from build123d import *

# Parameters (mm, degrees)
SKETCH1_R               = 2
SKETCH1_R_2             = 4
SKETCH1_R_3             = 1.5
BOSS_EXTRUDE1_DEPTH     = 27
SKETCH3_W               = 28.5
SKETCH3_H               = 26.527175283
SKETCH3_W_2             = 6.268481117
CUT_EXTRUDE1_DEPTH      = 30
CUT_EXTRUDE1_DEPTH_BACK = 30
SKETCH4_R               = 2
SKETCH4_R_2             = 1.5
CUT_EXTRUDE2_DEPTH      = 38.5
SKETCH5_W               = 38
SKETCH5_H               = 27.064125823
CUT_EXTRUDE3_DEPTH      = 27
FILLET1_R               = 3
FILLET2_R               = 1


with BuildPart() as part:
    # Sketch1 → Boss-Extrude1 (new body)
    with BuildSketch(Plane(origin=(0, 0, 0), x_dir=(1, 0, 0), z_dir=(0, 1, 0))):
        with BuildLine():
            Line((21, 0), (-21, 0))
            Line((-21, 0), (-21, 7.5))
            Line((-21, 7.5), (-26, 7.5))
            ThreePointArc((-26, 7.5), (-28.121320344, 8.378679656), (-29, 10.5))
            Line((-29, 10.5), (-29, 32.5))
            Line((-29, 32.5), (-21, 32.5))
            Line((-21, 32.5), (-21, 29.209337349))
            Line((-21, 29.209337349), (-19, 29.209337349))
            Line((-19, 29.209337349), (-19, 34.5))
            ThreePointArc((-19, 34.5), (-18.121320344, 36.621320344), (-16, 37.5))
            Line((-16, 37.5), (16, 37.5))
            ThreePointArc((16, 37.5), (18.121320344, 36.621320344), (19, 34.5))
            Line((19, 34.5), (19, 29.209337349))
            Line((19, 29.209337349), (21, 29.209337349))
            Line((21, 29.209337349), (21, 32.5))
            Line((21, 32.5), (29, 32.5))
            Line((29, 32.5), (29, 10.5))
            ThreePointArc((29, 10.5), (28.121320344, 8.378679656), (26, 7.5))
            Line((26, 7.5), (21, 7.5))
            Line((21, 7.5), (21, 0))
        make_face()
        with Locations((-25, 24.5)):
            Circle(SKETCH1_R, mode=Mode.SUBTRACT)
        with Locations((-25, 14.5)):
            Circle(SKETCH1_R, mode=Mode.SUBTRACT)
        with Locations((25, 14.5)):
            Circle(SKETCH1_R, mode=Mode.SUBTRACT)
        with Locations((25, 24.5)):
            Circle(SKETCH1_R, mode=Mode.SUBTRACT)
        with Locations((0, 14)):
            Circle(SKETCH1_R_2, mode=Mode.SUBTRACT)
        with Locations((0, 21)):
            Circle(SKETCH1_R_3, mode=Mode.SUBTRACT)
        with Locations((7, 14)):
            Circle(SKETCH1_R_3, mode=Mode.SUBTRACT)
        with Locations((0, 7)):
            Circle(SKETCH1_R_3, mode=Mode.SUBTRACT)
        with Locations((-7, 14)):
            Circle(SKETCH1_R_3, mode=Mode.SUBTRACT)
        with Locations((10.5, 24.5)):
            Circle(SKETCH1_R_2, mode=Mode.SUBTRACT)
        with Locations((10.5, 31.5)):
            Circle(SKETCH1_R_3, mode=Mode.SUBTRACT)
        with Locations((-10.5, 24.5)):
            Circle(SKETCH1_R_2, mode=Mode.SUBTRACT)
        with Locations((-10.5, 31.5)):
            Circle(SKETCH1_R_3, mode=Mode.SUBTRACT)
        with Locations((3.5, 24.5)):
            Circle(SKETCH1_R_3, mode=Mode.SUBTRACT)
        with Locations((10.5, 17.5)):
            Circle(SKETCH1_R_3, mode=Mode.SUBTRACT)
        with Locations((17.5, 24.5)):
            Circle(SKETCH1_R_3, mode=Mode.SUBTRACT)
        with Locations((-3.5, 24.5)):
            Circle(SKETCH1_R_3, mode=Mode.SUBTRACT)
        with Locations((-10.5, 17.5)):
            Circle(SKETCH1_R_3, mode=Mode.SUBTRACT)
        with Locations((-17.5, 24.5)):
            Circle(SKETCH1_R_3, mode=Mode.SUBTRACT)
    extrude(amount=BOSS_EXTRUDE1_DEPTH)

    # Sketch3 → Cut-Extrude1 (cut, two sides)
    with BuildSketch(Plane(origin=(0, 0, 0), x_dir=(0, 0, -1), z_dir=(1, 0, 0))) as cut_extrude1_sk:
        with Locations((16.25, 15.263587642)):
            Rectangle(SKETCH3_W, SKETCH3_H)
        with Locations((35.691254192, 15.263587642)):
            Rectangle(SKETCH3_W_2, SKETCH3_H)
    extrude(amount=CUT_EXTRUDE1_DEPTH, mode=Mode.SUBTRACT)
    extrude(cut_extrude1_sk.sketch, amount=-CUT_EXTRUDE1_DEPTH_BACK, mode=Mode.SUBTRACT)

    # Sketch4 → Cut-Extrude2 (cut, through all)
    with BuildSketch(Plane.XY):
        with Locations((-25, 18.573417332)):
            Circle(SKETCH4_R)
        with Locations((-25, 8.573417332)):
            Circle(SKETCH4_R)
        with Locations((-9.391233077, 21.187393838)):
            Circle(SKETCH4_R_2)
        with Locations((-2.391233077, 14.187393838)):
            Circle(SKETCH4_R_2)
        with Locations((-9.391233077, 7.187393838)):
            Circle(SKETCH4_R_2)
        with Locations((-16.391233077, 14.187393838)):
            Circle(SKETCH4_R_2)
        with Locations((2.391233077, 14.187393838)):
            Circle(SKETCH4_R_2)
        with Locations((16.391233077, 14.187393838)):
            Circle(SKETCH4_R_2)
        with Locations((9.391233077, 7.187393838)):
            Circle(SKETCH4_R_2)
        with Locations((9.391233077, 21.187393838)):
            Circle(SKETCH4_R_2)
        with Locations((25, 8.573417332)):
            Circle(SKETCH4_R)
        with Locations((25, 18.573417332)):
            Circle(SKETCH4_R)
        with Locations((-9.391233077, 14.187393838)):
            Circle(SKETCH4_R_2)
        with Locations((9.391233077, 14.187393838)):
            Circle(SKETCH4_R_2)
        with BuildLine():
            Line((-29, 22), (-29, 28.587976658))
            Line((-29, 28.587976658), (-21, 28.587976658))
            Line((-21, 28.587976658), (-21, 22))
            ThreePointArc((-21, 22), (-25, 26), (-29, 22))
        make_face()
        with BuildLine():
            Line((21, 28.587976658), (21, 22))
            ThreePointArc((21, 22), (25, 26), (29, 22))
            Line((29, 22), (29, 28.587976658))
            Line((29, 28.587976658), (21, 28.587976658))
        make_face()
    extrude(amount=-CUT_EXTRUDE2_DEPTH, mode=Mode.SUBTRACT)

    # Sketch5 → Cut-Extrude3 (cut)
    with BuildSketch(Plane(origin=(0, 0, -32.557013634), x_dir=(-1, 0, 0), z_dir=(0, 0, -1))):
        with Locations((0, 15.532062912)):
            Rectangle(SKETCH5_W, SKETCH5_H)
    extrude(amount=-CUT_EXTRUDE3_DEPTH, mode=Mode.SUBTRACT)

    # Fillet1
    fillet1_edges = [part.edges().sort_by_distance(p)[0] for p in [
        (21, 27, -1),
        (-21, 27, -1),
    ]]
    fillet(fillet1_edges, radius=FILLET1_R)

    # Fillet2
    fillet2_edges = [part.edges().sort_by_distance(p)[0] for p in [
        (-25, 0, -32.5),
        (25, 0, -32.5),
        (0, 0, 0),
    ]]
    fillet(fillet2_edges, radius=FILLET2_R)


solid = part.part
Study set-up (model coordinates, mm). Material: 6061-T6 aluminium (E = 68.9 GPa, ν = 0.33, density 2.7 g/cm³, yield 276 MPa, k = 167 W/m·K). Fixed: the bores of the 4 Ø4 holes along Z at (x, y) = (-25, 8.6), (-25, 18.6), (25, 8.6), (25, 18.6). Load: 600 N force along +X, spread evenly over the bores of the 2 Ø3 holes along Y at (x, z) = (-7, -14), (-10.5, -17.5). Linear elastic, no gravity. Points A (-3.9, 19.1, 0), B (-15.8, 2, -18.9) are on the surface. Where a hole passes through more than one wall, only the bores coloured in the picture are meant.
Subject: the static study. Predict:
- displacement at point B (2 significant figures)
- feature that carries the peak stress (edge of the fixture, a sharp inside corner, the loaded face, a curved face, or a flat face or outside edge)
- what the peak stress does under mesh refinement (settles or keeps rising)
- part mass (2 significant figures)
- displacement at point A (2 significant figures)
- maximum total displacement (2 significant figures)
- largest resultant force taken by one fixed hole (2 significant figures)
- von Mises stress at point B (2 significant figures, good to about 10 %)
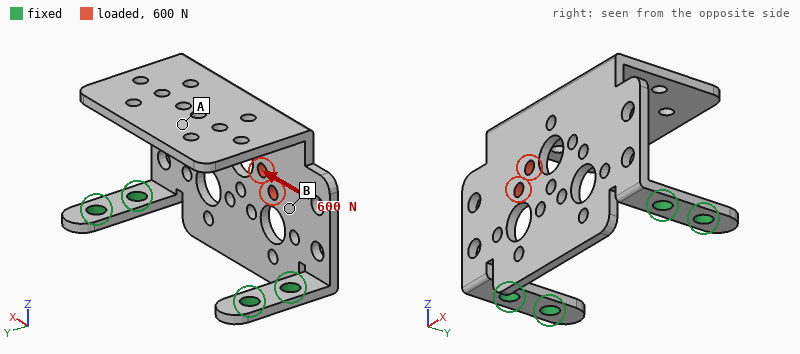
0.059 mm
edge of the fixture
keeps rising
16 g
0.12 mm
0.15 mm
390 N
31 MPa
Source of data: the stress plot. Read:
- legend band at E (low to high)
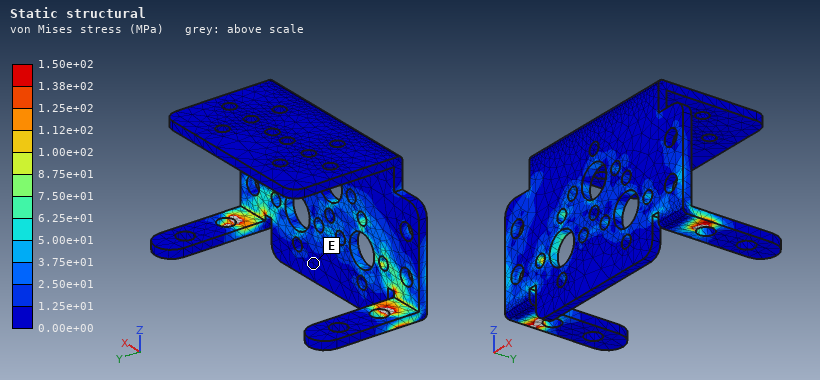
0.00e+00 to 1.25e+01 MPa
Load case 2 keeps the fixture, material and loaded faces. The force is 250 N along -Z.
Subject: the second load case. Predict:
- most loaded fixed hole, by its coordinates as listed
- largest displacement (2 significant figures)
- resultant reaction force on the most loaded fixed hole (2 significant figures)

(-25, 8.6)
0.24 mm
170 N
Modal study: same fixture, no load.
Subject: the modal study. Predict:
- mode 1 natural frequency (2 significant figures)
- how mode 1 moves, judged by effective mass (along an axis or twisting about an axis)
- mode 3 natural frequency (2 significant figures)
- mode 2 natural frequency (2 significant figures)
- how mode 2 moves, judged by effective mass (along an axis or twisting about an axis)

390 Hz
along Y
1500 Hz
1200 Hz
along X
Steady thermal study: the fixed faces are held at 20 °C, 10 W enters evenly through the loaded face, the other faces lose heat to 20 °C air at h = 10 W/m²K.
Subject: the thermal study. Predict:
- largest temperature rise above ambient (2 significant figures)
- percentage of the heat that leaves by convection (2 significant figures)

43 K
18 %
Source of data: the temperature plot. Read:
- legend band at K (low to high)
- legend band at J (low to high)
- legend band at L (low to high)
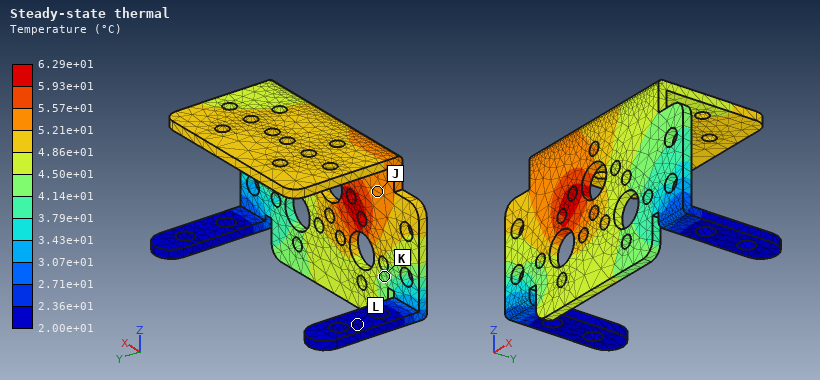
4.14e+01 to 4.50e+01 °C
5.21e+01 to 5.57e+01 °C
2.00e+01 to 2.36e+01 °C
